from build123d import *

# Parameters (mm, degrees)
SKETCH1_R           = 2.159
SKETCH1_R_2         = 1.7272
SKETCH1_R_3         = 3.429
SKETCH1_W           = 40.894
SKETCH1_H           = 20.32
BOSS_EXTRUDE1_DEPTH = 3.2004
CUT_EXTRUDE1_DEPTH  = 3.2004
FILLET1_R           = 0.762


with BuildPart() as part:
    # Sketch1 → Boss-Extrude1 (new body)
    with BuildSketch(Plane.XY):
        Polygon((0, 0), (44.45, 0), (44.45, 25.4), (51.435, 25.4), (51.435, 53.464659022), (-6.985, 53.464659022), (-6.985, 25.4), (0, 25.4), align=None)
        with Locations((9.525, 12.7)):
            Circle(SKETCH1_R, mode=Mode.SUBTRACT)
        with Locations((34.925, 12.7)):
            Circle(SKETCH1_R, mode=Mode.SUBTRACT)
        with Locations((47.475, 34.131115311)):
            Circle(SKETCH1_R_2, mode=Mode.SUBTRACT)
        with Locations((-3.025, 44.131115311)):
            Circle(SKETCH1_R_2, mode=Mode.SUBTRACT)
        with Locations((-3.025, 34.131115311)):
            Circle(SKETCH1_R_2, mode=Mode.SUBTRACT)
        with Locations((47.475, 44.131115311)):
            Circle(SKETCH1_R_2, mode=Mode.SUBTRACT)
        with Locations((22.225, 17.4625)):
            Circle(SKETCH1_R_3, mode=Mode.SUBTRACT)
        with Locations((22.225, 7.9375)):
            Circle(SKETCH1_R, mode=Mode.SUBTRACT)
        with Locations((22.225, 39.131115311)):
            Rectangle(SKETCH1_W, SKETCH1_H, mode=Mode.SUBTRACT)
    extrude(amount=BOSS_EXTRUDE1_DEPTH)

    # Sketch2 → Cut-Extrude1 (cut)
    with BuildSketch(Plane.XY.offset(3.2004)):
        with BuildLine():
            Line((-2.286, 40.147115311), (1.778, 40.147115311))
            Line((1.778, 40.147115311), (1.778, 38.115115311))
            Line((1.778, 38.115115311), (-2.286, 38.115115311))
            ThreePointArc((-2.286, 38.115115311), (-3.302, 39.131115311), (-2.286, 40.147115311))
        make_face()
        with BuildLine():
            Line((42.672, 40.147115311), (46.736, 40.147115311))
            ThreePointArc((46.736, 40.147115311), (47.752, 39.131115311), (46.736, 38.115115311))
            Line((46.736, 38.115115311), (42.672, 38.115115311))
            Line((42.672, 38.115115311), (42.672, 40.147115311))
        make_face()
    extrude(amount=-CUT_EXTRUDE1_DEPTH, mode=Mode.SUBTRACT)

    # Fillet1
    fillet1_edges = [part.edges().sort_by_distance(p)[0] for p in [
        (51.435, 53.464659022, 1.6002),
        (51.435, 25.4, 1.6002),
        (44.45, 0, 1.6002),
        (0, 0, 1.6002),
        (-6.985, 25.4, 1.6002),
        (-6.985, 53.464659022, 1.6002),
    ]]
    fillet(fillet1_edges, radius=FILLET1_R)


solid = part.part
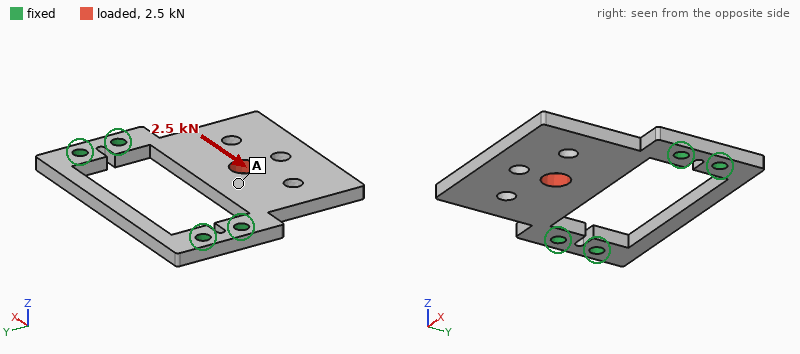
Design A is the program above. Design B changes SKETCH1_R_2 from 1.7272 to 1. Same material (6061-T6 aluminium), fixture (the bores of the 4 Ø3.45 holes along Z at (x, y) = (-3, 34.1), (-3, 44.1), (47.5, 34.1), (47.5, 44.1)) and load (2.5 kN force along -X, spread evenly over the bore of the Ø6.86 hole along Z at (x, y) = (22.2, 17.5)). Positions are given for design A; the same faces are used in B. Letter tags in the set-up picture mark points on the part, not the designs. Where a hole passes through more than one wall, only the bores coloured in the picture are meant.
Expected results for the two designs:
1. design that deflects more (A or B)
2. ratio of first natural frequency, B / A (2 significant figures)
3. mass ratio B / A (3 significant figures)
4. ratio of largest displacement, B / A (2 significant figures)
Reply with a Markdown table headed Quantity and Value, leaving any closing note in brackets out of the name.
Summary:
| Quantity | Value |
|---|---|
| design that deflects more | B |
| ratio of first natural frequency, B / A | 0.95 |
| mass ratio B / A | 1.01 |
| ratio of largest displacement, B / A | 1.2 |
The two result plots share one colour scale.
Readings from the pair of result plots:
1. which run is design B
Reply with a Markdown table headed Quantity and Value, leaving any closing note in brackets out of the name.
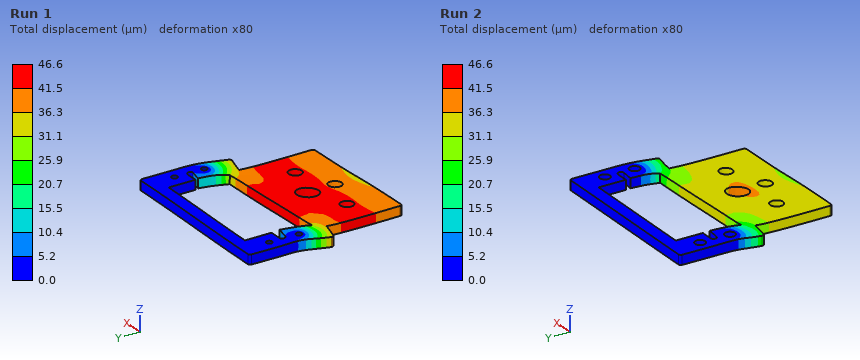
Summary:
| Quantity | Value |
|---|---|
| which run is design B | Run 1 |
